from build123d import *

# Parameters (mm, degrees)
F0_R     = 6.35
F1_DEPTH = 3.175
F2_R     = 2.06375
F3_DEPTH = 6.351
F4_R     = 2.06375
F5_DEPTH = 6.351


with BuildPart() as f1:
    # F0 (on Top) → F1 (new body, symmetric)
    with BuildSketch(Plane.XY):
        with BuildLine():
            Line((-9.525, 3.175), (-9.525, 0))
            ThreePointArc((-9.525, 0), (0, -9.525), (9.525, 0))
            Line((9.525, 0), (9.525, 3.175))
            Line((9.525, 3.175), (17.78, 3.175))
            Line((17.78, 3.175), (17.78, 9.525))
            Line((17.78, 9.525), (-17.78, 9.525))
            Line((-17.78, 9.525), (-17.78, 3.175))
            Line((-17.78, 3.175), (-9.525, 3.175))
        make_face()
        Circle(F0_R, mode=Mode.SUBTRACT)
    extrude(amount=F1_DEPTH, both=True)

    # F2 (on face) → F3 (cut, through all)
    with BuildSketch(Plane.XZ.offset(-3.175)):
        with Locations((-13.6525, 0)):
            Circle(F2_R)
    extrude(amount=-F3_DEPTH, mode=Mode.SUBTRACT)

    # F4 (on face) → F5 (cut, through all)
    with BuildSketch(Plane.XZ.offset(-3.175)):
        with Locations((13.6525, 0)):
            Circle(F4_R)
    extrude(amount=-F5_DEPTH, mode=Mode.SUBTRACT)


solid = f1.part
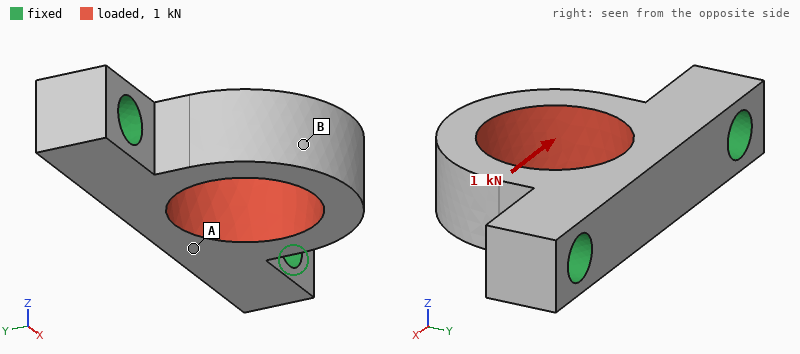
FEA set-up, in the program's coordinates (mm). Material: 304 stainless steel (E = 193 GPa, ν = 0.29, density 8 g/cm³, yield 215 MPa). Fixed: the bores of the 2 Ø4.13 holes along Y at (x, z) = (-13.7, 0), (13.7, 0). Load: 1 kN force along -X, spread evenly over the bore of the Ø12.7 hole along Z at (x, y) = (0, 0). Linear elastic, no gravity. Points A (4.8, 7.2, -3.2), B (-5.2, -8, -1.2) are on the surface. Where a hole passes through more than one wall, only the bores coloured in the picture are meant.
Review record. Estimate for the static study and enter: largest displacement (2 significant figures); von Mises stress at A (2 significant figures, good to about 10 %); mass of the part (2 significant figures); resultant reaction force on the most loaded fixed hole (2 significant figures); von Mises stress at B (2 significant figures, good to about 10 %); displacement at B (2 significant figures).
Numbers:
8.3 µm
10 MPa
14 g
550 N
34 MPa
7.9 µm
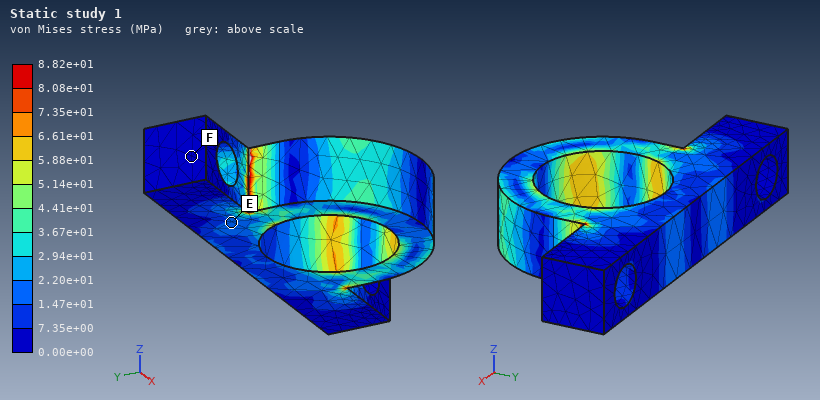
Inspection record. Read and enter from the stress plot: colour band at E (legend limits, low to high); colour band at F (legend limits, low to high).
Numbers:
1.47e+01 to 2.20e+01 MPa
0.00e+00 to 7.35e+00 MPa
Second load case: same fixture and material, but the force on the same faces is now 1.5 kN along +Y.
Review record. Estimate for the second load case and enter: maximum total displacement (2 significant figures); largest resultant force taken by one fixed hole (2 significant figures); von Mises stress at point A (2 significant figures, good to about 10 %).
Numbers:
3.8 µm
750 N
13 MPa
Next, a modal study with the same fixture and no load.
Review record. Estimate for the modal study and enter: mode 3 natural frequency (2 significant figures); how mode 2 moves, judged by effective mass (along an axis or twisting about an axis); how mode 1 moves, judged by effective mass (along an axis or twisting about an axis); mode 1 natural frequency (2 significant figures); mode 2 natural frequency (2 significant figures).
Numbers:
30 kHz
along X
along Z
13 kHz
21 kHz
